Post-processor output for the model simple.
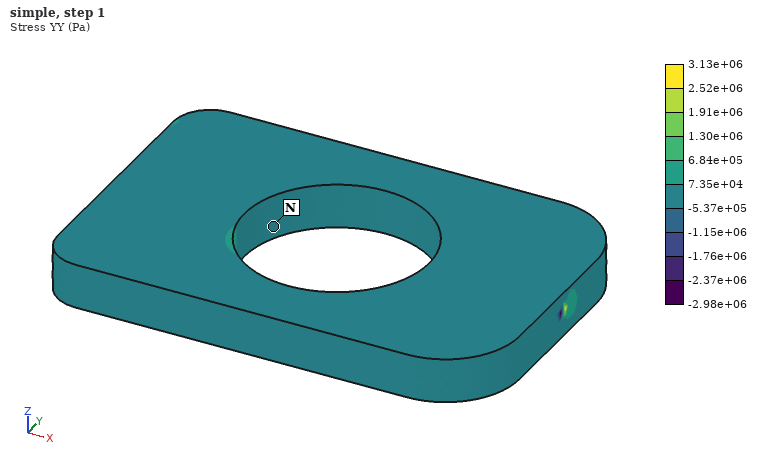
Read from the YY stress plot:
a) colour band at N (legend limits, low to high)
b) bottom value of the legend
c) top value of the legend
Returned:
-5.37e+05 to 7.35e+04 Pa
-2.98e+06 Pa
3.13e+06 Pa
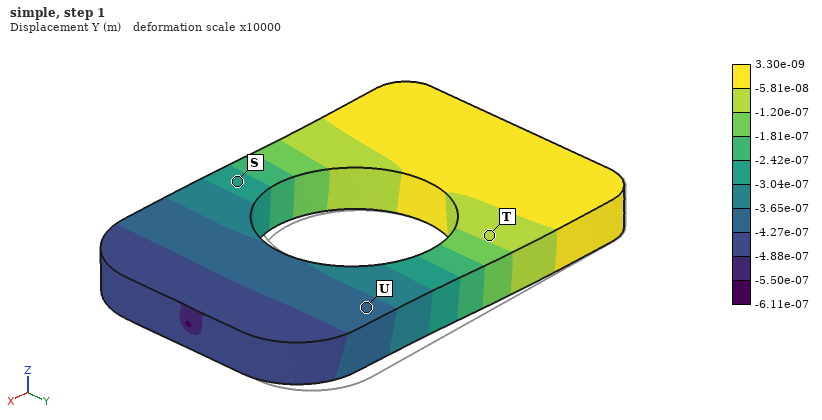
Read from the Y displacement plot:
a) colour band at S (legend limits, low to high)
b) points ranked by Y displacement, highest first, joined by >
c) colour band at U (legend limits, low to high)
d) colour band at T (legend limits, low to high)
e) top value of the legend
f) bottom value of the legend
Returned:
-3.04e-07 to -2.42e-07 m
T > S > U
-4.27e-07 to -3.65e-07 m
-1.20e-07 to -5.81e-08 m
3.30e-09 m
-6.11e-07 m
